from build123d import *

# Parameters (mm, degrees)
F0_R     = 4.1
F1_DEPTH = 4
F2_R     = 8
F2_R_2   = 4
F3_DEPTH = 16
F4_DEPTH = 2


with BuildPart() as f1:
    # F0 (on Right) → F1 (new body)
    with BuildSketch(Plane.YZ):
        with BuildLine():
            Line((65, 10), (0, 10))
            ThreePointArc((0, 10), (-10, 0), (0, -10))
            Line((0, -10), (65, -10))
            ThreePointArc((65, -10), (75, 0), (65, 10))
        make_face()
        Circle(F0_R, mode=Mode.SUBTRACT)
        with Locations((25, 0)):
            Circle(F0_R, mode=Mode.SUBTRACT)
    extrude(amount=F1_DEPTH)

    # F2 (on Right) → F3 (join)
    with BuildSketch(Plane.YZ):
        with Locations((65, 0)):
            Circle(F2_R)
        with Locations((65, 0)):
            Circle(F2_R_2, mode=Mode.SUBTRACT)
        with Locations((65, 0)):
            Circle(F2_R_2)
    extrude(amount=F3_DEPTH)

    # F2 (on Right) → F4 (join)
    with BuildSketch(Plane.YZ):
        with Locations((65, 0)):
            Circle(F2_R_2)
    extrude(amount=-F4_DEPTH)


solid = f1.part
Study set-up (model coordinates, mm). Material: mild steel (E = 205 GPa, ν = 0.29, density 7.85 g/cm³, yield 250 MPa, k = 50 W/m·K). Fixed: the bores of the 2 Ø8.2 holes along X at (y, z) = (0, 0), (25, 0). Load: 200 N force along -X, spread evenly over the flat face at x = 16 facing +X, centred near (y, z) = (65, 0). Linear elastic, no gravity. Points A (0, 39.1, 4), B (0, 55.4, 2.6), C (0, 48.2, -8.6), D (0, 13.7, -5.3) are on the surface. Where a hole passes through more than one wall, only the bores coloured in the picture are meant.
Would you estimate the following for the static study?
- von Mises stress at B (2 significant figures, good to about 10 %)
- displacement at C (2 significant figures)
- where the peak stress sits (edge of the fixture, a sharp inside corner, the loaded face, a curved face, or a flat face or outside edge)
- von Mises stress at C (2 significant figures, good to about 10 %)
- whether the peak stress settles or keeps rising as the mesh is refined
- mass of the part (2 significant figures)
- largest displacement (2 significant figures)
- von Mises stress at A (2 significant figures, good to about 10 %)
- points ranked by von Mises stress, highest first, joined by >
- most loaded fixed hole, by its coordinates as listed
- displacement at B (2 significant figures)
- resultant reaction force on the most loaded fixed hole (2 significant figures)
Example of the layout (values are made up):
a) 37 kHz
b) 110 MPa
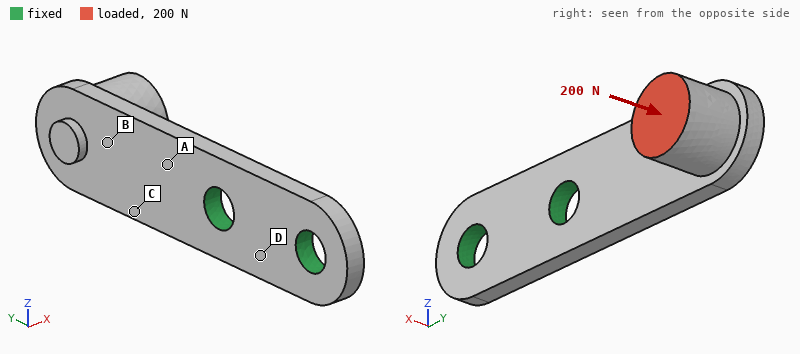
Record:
a) 35 MPa
b) 0.058 mm
c) edge of the fixture
d) 64 MPa
e) keeps rising
f) 67 g
g) 0.22 mm
h) 91 MPa
i) A > C > B > D
j) (25, 0)
k) 0.098 mm
l) 200 N
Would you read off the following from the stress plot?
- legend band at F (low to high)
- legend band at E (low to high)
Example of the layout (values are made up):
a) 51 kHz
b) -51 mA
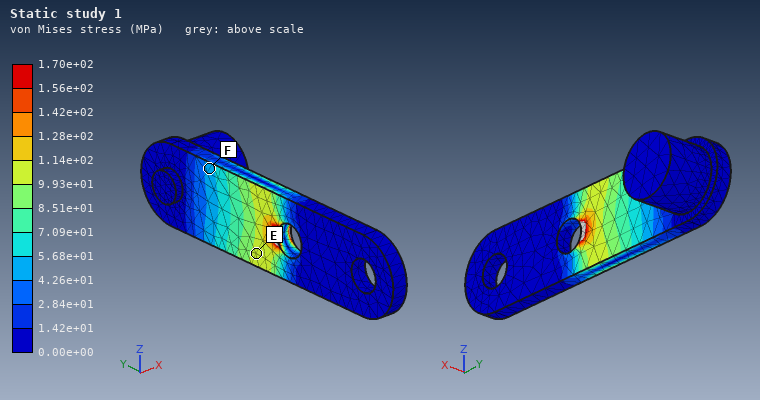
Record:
a) 4.26e+01 to 5.68e+01 MPa
b) 9.93e+01 to 1.14e+02 MPa
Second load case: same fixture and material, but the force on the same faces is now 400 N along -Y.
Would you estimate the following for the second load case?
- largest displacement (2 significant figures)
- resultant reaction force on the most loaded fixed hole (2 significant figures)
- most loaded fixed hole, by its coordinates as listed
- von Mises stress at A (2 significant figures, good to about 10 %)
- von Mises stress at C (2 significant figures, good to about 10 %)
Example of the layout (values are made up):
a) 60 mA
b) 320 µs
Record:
a) 0.26 mm
b) 380 N
c) (25, 0)
d) 95 MPa
e) 100 MPa
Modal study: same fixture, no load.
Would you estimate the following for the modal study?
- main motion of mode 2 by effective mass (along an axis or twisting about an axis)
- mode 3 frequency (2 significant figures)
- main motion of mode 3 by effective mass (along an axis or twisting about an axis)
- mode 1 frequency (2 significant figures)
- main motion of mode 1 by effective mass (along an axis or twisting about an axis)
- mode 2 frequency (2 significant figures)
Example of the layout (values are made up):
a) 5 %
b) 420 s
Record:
a) along Z
b) 5300 Hz
c) along Z
d) 970 Hz
e) along X
f) 2900 Hz
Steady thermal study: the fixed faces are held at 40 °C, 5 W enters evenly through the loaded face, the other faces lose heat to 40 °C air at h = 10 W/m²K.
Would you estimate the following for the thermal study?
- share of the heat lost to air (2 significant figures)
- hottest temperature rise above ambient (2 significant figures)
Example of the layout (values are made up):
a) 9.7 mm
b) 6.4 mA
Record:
a) 15 %
b) 44 K
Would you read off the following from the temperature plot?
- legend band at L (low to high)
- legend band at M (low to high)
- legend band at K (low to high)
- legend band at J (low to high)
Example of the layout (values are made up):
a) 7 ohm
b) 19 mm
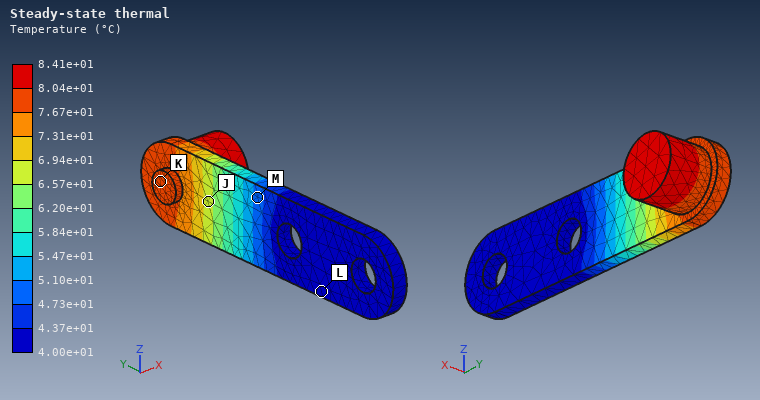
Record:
a) 4.00e+01 to 4.37e+01 °C
b) 4.73e+01 to 5.10e+01 °C
c) 7.67e+01 to 8.04e+01 °C
d) 6.57e+01 to 6.94e+01 °C
